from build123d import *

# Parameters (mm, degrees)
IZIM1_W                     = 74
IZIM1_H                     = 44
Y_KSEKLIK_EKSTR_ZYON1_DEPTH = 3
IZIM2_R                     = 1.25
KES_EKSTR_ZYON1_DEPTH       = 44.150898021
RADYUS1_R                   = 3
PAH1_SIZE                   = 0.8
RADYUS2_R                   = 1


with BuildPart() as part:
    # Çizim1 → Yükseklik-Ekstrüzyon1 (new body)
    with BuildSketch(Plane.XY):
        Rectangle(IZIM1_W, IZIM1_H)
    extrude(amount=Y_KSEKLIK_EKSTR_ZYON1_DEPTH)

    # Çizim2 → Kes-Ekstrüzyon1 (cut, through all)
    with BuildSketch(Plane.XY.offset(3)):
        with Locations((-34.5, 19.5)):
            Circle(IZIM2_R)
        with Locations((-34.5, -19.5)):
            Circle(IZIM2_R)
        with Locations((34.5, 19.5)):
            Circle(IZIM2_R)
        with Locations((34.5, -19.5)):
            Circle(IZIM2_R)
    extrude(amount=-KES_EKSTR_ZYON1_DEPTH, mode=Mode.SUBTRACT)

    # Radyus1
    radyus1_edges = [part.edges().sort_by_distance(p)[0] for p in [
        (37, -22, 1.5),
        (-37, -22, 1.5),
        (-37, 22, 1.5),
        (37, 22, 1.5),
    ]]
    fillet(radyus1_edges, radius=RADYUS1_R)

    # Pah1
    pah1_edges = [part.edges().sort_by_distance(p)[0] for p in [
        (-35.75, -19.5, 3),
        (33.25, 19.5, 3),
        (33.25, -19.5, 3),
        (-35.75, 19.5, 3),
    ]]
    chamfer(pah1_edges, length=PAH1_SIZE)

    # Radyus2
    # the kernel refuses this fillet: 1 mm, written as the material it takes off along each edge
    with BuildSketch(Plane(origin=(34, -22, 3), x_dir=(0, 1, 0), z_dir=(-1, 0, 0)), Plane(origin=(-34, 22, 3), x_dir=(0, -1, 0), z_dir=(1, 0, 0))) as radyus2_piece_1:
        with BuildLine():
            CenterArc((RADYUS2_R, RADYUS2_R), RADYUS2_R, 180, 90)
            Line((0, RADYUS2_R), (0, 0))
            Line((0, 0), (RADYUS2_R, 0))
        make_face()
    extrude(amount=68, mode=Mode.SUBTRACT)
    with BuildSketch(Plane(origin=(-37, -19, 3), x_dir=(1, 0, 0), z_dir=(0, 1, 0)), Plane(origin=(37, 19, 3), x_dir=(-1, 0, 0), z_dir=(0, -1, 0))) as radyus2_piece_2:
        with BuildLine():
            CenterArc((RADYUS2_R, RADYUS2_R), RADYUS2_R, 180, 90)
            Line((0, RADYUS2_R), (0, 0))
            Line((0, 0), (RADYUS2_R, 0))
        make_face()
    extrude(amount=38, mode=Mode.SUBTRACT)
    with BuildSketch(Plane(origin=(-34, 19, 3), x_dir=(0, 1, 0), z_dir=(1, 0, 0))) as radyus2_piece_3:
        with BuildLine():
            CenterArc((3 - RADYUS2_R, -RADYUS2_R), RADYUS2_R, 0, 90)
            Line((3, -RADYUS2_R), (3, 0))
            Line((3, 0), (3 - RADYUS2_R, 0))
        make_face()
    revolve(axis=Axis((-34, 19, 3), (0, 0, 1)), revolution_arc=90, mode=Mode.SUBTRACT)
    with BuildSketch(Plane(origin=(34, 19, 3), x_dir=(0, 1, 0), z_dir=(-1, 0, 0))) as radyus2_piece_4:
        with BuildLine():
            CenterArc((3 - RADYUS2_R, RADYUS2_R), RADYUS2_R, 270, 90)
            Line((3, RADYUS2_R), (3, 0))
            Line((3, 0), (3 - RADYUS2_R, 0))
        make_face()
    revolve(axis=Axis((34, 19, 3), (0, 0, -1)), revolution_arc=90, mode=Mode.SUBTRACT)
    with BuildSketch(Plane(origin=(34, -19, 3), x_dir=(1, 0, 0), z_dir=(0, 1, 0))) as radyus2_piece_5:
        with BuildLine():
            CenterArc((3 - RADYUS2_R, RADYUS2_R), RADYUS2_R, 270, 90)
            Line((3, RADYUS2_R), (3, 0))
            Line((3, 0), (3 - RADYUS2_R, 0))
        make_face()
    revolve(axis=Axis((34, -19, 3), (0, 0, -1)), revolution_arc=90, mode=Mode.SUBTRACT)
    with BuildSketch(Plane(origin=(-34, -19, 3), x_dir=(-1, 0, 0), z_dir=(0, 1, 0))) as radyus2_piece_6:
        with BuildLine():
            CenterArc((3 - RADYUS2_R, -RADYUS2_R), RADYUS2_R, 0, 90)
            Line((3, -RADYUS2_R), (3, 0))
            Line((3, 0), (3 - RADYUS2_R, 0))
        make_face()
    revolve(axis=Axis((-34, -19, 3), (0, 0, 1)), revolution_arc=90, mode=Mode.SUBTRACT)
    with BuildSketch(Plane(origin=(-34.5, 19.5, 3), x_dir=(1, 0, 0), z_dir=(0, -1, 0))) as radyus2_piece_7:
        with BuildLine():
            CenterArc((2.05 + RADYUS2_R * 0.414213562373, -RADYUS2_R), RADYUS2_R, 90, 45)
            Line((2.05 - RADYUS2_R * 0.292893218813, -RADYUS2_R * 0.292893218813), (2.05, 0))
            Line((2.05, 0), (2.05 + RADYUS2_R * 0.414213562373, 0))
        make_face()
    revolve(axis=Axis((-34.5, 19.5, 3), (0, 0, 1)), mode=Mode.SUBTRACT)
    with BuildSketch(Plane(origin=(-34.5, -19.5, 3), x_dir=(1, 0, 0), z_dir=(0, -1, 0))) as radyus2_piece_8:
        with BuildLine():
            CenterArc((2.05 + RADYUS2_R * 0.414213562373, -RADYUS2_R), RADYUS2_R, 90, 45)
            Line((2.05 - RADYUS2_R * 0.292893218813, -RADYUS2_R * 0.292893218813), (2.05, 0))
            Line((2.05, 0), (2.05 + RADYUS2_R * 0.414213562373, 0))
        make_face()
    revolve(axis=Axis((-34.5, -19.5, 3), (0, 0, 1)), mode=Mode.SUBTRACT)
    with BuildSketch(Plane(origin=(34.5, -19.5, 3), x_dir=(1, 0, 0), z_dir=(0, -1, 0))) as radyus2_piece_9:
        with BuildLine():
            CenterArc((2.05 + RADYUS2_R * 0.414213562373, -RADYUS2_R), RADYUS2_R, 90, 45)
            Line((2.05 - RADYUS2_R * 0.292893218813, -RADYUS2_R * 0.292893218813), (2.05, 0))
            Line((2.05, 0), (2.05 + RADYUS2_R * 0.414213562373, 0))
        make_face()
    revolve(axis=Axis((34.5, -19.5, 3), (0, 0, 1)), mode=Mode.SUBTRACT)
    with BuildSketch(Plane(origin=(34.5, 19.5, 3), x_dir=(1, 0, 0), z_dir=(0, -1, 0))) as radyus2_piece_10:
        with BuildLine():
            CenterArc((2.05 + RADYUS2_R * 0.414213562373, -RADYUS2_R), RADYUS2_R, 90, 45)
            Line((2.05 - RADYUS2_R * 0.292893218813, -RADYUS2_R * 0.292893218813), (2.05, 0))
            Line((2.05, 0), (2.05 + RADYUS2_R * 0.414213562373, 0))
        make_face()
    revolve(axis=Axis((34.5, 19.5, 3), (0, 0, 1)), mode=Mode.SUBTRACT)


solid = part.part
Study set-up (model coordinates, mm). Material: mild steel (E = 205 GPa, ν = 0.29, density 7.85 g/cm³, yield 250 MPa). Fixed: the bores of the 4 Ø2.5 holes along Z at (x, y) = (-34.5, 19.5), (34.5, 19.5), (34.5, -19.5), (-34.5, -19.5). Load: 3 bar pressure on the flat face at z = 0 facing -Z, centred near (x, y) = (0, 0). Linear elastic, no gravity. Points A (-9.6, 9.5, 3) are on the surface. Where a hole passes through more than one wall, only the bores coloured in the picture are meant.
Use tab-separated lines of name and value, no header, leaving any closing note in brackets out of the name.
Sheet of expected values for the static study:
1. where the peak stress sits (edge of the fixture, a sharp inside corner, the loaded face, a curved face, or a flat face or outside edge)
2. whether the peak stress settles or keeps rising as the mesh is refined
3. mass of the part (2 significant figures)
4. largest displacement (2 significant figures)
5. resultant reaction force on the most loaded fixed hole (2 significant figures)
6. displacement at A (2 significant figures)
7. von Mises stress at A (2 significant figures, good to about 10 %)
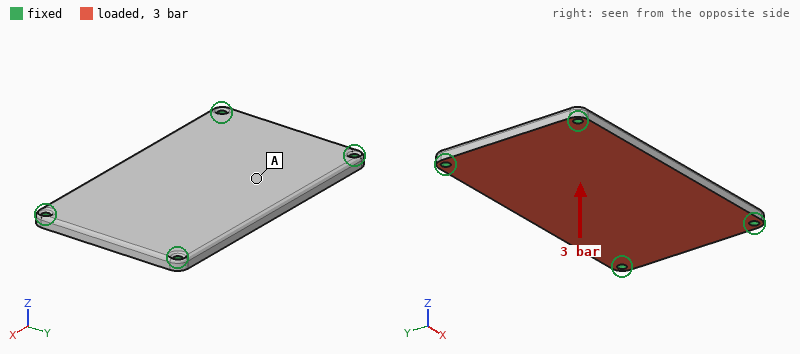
where the peak stress sits	edge of the fixture
whether the peak stress settles or keeps rising as the mesh is refined	keeps rising
mass of the part	76 g
largest displacement	69 µm
resultant reaction force on the most loaded fixed hole	260 N
displacement at A	61 µm
von Mises stress at A	43 MPa
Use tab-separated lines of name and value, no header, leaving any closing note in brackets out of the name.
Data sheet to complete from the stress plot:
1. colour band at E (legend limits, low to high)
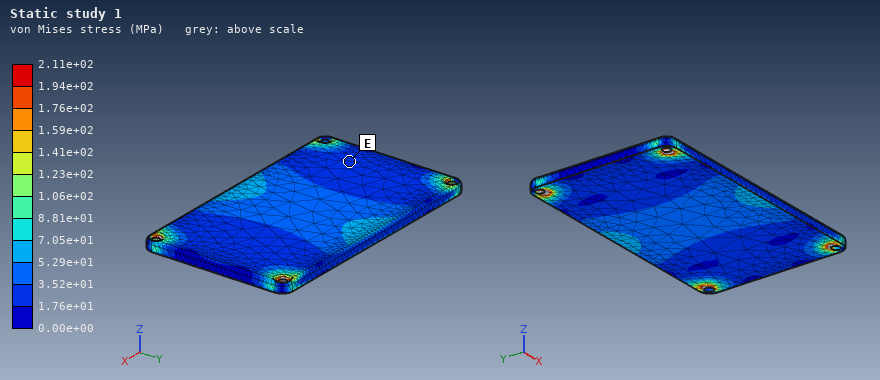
colour band at E	1.76e+01 to 3.52e+01 MPa
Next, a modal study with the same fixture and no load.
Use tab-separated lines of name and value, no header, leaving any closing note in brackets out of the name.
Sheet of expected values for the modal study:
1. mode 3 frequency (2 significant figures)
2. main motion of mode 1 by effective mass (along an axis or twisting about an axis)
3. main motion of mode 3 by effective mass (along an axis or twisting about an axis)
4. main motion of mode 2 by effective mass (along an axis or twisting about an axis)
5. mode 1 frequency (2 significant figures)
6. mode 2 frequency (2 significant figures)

mode 3 frequency	6600 Hz
main motion of mode 1 by effective mass	along Z
main motion of mode 3 by effective mass	twisting about Y
main motion of mode 2 by effective mass	twisting about X
mode 1 frequency	2500 Hz
mode 2 frequency	4500 Hz
